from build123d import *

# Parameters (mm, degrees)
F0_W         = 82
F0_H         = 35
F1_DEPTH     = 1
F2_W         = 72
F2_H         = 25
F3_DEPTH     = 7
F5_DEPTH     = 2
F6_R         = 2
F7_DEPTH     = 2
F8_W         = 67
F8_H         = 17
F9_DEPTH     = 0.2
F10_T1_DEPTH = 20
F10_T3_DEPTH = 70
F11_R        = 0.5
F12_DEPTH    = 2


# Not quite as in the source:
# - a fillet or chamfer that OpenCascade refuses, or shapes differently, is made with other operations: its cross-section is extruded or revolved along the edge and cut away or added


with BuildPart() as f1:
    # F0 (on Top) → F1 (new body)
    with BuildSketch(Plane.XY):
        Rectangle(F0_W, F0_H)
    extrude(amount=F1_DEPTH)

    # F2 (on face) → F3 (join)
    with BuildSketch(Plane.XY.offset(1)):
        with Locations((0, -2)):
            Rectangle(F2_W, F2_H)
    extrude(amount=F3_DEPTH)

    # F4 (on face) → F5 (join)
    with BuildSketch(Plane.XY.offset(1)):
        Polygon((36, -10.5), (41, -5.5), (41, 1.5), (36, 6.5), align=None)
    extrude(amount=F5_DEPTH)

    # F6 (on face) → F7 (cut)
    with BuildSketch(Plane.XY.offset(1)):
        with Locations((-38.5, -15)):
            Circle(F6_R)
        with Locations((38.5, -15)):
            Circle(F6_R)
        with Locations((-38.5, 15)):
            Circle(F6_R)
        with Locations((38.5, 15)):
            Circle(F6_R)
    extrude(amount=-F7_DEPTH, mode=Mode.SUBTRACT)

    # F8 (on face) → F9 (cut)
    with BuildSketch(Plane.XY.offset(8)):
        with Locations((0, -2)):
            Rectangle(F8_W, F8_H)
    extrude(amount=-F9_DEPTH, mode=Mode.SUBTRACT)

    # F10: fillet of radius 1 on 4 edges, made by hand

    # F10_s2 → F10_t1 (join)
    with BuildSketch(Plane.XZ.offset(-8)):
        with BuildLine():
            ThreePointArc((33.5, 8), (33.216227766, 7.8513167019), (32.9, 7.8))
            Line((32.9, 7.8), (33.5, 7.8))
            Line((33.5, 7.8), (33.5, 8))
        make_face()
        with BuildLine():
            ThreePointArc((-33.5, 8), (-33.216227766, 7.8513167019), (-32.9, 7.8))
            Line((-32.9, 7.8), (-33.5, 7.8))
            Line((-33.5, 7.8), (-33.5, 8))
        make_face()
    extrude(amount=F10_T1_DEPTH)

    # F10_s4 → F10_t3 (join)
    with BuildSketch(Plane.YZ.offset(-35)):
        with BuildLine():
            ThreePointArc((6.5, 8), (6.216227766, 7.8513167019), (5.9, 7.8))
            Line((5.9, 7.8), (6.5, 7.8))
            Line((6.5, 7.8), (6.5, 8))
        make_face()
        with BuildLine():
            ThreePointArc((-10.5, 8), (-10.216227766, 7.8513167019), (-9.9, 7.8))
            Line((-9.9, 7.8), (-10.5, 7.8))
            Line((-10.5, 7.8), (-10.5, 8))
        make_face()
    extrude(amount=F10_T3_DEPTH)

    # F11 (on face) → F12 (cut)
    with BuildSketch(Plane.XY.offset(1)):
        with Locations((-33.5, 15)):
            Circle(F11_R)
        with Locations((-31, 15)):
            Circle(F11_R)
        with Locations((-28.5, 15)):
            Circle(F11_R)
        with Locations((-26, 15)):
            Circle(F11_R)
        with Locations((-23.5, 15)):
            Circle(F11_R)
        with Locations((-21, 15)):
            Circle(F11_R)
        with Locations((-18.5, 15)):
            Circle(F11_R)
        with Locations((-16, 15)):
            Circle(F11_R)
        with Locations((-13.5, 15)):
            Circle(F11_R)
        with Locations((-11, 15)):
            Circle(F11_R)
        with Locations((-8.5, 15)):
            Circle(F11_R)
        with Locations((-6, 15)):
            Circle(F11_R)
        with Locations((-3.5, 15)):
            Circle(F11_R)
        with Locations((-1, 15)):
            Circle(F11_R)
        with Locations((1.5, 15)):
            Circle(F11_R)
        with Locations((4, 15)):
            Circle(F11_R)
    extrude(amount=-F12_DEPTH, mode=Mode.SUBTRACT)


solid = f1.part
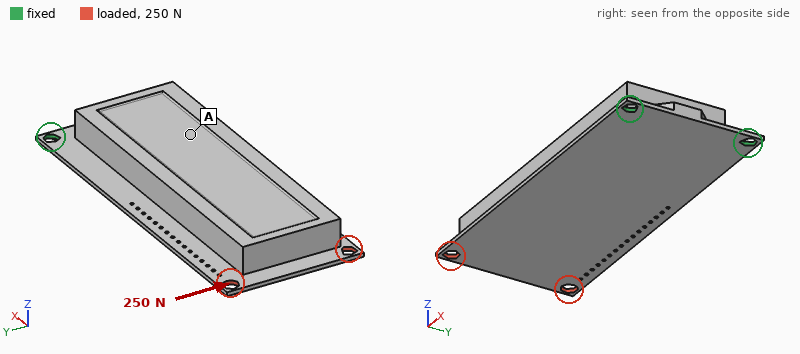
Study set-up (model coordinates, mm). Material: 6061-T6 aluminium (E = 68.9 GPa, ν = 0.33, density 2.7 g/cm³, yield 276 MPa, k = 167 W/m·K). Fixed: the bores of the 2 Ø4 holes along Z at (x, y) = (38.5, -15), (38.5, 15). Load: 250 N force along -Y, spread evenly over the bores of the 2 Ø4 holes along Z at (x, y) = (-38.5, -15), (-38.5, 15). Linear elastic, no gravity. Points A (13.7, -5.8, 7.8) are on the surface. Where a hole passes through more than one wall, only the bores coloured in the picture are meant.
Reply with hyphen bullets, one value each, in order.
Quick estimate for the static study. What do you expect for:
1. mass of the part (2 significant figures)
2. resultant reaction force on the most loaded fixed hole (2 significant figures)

- 41 g
- 670 N
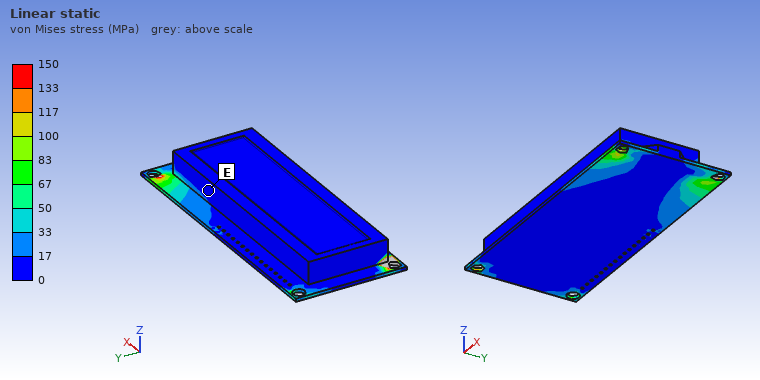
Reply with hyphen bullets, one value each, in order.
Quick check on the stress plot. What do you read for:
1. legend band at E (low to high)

- 0 to 17 MPa
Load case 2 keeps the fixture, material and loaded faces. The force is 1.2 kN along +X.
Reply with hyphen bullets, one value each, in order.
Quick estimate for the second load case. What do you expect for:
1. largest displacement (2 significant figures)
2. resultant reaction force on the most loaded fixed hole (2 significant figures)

- 0.17 mm
- 650 N
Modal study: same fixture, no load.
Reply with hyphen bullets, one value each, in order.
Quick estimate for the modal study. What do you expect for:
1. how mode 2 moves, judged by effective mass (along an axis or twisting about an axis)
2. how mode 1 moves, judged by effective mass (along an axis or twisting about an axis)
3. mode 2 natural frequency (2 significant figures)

- along Y
- along Z
- 2500 Hz
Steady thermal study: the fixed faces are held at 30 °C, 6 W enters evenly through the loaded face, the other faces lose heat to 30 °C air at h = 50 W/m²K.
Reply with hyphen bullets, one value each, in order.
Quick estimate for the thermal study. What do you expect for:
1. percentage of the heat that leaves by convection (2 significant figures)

- 50 %
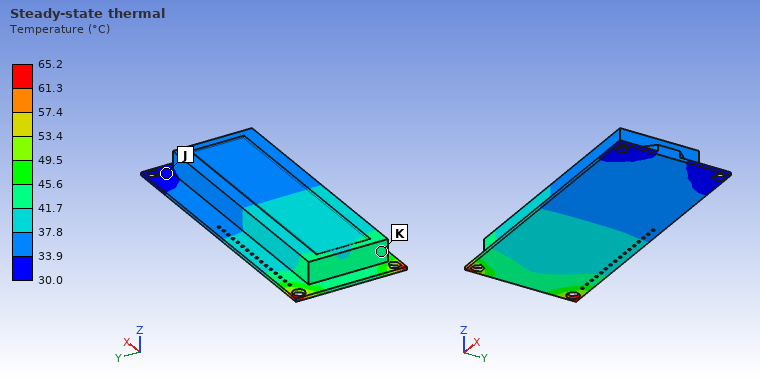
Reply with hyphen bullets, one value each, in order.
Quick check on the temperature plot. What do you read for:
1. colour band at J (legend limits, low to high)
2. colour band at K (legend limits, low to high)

- 30.0 to 33.9 °C
- 41.7 to 45.6 °C
